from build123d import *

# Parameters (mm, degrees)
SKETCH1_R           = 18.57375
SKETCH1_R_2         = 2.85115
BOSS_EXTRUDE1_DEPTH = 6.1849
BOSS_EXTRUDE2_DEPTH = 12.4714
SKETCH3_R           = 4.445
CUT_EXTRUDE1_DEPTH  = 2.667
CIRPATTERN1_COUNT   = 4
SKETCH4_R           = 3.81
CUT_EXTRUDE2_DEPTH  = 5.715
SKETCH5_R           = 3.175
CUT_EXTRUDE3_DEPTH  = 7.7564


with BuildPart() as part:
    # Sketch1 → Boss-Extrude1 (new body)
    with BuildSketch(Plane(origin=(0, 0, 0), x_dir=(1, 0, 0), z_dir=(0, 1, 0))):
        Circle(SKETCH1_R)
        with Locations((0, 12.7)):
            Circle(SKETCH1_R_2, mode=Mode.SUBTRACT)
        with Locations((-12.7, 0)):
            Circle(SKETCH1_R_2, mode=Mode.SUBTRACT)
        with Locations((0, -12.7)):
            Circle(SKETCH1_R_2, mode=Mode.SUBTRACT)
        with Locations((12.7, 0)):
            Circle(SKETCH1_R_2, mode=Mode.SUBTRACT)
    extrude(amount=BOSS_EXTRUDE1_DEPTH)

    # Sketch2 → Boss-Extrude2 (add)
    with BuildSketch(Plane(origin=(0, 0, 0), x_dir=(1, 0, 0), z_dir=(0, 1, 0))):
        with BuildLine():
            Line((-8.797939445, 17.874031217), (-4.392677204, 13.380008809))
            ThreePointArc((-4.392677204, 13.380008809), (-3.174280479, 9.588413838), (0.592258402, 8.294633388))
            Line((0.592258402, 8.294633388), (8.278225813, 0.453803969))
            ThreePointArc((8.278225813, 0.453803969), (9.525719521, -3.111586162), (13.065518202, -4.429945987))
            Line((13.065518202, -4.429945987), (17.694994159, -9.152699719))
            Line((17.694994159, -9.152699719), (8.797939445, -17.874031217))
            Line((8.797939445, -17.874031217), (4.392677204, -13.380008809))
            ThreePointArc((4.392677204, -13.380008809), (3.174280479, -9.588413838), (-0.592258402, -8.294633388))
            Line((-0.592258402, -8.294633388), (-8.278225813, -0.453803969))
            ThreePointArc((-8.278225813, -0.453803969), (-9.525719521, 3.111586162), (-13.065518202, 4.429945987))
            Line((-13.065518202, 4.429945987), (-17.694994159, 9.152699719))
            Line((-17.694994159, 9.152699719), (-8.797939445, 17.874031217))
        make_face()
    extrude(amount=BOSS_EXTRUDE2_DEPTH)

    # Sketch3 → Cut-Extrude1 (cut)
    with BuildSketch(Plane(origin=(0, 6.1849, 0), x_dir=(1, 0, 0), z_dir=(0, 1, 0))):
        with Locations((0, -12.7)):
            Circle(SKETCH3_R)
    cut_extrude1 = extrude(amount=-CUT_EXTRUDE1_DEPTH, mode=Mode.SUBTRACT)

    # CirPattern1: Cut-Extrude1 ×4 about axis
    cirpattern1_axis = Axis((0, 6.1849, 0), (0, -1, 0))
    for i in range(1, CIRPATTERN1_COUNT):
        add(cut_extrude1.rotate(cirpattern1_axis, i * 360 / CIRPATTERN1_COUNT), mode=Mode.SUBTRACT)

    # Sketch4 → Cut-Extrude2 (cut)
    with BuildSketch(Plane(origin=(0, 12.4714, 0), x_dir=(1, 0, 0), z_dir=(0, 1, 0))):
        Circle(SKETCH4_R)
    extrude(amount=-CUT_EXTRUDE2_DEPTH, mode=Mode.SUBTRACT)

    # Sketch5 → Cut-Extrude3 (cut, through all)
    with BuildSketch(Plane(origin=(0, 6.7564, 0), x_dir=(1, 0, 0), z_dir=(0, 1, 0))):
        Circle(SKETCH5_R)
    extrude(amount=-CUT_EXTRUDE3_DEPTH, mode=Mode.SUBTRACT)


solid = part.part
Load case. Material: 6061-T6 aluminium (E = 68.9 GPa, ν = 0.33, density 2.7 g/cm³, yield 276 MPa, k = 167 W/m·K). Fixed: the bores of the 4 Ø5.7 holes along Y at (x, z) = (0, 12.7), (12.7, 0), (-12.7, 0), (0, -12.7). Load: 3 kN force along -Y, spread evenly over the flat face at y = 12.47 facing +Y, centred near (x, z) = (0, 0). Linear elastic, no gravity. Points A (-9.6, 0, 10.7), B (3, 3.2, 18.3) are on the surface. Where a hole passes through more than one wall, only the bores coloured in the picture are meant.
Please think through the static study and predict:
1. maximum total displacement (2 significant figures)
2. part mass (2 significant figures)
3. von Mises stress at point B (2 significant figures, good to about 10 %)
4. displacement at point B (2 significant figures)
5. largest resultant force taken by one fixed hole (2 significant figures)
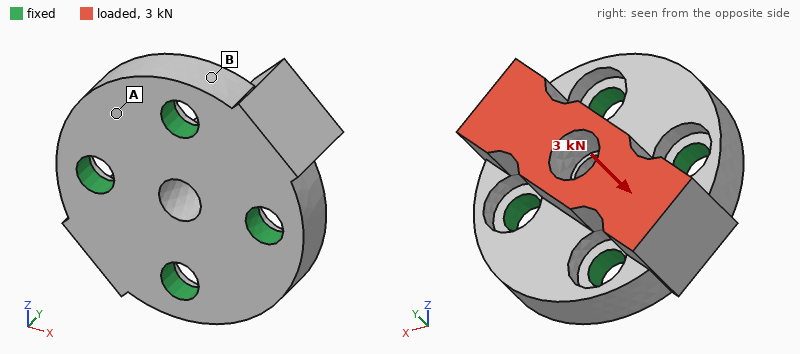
6.1 µm
22 g
11 MPa
1.5 µm
800 N
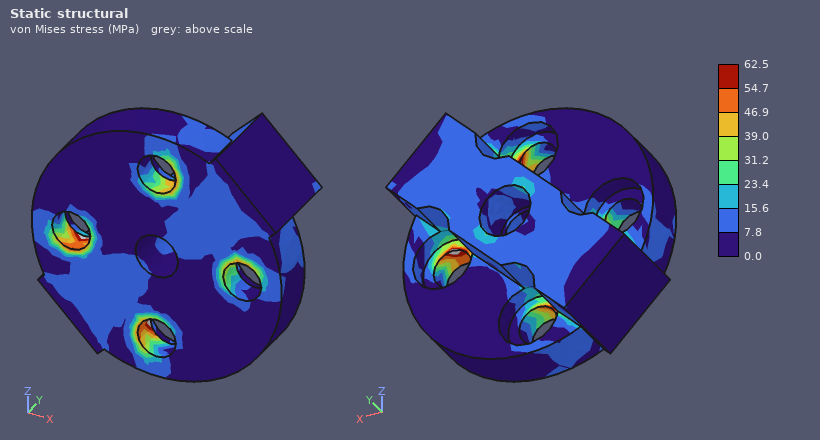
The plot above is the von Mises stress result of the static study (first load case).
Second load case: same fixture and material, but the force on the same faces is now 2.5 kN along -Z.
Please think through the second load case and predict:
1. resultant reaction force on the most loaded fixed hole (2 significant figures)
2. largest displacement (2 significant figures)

1.2 kN
13 µm
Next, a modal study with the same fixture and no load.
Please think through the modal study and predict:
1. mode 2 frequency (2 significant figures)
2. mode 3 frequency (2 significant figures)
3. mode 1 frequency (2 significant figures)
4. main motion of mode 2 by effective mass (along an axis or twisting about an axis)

35 kHz
39 kHz
29 kHz
along Y
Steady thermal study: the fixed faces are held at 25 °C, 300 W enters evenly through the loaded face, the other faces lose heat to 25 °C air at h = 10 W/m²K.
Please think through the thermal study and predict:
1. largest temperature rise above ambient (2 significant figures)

71 K
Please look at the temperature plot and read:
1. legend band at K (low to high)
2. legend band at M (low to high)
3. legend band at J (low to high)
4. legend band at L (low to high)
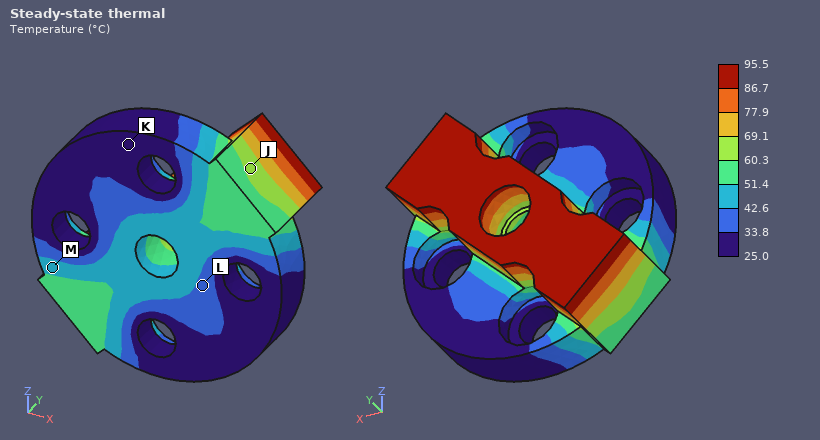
25.0 to 33.8 °C
42.6 to 51.4 °C
60.3 to 69.1 °C
33.8 to 42.6 °C
